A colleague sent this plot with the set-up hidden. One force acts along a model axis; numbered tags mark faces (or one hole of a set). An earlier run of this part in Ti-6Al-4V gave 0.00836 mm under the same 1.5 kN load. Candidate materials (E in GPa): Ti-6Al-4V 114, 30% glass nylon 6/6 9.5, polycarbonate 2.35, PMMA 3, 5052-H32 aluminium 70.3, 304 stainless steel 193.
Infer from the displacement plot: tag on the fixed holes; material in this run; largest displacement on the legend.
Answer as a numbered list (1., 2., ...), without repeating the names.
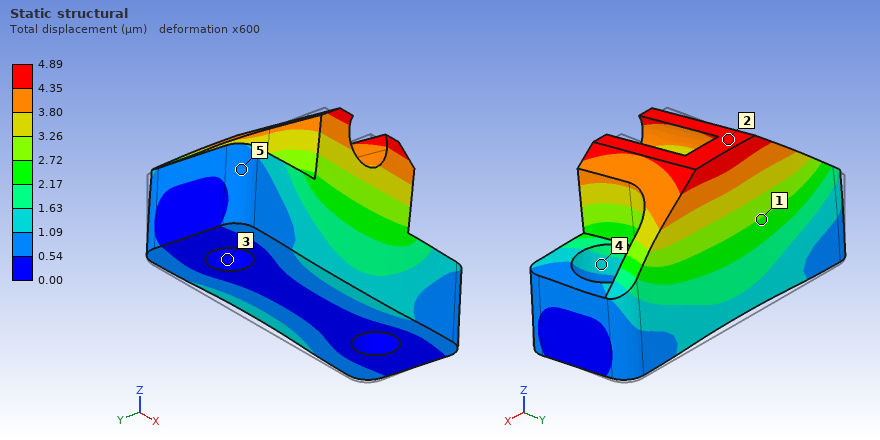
1. 3
2. 304 stainless steel
3. 4.89 µm
